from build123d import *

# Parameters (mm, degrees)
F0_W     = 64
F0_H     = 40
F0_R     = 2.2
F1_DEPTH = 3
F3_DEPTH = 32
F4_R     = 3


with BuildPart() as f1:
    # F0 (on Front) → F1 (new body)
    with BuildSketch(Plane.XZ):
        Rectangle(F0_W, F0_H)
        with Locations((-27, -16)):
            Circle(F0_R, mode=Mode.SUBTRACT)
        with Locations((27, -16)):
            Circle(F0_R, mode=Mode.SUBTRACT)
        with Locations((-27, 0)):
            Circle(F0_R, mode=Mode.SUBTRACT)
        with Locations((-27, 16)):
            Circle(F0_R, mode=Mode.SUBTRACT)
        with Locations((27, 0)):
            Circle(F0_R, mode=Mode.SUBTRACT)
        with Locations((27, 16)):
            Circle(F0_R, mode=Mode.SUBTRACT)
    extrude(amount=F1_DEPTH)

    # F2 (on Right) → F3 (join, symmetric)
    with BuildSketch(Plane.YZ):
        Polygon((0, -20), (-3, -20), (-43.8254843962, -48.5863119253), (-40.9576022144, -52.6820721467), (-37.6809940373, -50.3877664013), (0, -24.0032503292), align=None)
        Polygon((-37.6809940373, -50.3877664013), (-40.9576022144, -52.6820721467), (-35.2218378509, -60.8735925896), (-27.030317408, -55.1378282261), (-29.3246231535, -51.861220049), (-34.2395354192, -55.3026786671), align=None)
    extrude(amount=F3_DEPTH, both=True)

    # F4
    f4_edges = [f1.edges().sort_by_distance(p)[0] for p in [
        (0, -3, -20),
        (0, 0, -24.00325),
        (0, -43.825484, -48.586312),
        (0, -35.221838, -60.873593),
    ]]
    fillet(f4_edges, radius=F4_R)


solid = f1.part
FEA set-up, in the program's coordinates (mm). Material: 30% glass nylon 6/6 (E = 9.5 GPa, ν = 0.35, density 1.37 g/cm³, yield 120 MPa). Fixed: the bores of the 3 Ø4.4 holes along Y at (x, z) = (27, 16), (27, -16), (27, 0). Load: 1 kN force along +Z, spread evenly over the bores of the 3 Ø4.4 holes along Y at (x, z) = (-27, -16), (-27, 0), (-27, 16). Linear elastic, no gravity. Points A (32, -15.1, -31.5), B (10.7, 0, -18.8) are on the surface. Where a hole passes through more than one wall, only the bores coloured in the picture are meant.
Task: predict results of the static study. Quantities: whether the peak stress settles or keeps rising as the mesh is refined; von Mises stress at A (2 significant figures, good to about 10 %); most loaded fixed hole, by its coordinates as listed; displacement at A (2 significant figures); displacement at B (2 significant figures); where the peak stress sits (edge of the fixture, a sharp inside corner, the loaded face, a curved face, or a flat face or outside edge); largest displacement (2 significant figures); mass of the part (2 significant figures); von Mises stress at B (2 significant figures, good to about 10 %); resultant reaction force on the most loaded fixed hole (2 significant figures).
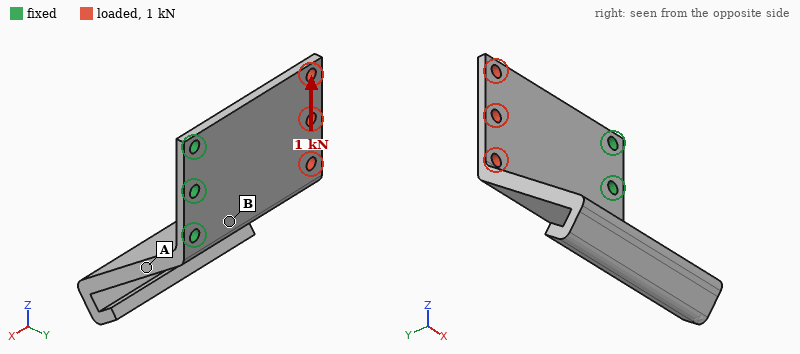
keeps rising
7.0 MPa
(27, -16)
0.11 mm
0.11 mm
edge of the fixture
0.48 mm
38 g
19 MPa
1.7 kN
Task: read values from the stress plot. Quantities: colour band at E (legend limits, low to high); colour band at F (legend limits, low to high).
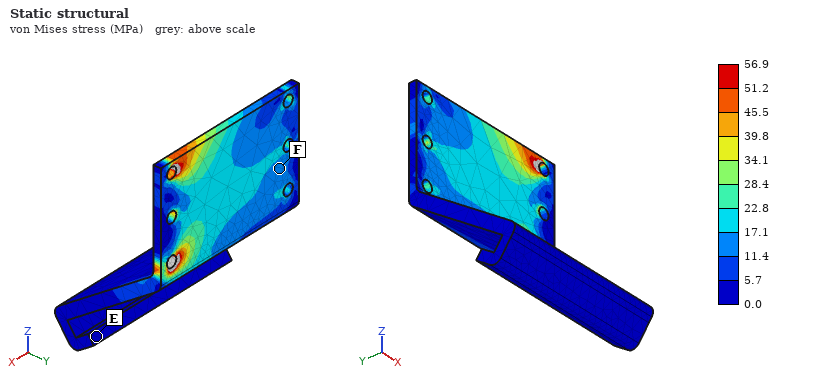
0.0 to 5.7 MPa
11.4 to 17.1 MPa
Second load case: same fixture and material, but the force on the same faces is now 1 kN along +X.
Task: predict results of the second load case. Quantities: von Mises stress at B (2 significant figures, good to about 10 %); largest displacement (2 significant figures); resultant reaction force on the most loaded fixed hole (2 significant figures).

3.9 MPa
73 µm
350 N
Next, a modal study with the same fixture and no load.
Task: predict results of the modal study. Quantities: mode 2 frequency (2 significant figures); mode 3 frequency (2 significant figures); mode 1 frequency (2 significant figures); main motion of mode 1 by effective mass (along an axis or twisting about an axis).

380 Hz
990 Hz
220 Hz
along Y
